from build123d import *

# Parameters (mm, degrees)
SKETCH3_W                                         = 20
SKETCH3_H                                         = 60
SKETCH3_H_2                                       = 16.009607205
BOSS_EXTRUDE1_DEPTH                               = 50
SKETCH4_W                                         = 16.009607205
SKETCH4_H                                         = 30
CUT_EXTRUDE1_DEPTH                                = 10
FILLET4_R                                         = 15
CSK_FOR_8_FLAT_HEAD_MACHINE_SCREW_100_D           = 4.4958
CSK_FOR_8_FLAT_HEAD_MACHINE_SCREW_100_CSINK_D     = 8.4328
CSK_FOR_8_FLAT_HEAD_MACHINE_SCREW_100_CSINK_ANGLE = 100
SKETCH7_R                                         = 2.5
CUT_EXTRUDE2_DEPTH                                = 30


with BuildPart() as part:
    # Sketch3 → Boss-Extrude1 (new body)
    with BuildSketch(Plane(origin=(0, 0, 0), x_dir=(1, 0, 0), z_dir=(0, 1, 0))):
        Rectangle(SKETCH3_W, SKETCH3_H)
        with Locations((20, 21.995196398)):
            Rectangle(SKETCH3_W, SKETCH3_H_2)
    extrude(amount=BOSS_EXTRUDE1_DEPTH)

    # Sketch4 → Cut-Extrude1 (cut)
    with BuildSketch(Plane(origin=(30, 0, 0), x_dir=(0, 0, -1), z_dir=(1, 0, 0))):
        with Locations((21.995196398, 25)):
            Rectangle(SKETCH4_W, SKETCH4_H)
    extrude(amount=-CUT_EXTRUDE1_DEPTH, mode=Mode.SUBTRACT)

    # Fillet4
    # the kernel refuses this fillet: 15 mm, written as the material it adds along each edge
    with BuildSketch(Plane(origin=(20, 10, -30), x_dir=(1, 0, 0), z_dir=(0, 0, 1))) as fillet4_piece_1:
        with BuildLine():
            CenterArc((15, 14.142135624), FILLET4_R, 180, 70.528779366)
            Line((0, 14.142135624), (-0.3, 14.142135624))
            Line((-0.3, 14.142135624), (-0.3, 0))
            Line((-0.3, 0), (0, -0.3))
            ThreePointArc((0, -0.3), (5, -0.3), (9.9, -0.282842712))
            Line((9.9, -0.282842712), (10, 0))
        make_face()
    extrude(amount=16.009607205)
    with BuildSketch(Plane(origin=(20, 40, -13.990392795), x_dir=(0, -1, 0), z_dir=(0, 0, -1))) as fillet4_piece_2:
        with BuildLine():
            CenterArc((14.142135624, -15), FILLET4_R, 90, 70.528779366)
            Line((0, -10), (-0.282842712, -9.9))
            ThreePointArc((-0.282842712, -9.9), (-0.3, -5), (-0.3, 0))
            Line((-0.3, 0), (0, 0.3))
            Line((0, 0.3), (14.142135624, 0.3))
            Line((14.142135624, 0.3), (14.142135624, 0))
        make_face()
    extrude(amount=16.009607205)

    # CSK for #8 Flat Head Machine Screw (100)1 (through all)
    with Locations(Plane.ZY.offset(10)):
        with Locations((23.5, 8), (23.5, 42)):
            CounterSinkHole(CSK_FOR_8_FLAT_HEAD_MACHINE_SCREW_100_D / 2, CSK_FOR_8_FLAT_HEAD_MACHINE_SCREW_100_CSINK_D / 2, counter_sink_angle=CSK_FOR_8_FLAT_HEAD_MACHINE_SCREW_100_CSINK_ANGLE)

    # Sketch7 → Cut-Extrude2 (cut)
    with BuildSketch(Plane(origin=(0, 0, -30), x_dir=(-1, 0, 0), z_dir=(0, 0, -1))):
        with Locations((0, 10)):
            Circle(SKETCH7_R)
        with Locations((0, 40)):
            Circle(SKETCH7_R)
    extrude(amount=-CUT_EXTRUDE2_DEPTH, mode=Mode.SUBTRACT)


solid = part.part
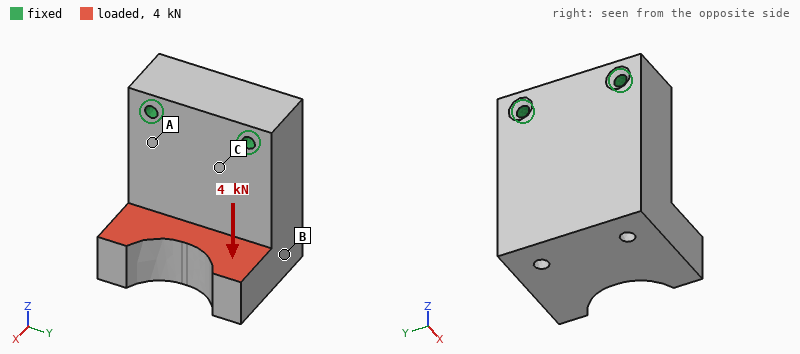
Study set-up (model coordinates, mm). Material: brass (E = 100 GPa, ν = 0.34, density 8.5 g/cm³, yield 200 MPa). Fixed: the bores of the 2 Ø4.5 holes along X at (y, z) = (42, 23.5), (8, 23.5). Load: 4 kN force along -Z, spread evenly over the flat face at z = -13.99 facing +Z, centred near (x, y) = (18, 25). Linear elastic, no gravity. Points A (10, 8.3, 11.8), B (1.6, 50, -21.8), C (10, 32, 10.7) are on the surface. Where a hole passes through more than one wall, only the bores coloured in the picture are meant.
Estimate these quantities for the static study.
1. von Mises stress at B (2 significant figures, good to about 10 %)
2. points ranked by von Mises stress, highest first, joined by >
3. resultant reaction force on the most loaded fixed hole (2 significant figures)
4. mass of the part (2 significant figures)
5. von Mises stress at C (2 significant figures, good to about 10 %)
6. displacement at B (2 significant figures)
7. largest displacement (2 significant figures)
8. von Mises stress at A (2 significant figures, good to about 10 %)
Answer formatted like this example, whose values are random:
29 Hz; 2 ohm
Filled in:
12 MPa; A > C > B; 2.0 kN; 600 g; 22 MPa; 29 µm; 57 µm; 32 MPa
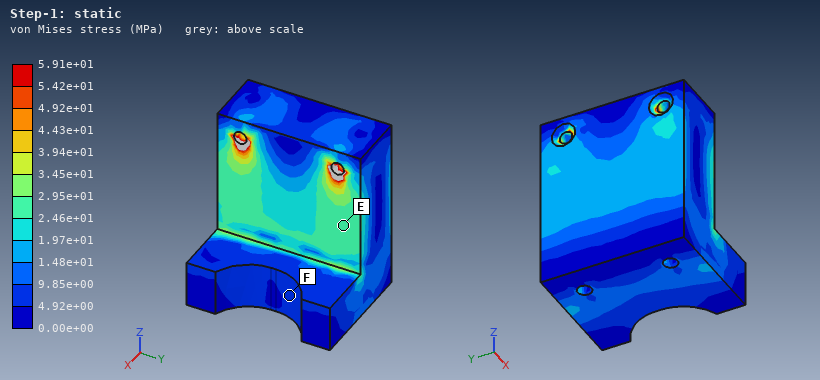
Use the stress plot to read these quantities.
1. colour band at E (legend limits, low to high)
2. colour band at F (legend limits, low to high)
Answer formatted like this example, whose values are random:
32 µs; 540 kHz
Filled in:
2.46e+01 to 2.95e+01 MPa; 4.92e+00 to 9.85e+00 MPa
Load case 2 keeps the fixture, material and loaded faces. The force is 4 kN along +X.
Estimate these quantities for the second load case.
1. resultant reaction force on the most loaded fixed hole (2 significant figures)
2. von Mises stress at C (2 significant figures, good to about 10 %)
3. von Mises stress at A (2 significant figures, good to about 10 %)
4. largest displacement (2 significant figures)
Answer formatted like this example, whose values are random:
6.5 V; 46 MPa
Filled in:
2.0 kN; 24 MPa; 39 MPa; 63 µm
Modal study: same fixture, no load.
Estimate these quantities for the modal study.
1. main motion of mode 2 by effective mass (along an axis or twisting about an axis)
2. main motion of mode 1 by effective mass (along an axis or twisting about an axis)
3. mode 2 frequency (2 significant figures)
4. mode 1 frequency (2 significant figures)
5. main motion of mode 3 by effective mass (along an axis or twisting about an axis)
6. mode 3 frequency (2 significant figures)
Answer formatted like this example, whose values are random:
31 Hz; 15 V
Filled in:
along Y; along X; 4200 Hz; 2300 Hz; along Y; 5700 Hz
